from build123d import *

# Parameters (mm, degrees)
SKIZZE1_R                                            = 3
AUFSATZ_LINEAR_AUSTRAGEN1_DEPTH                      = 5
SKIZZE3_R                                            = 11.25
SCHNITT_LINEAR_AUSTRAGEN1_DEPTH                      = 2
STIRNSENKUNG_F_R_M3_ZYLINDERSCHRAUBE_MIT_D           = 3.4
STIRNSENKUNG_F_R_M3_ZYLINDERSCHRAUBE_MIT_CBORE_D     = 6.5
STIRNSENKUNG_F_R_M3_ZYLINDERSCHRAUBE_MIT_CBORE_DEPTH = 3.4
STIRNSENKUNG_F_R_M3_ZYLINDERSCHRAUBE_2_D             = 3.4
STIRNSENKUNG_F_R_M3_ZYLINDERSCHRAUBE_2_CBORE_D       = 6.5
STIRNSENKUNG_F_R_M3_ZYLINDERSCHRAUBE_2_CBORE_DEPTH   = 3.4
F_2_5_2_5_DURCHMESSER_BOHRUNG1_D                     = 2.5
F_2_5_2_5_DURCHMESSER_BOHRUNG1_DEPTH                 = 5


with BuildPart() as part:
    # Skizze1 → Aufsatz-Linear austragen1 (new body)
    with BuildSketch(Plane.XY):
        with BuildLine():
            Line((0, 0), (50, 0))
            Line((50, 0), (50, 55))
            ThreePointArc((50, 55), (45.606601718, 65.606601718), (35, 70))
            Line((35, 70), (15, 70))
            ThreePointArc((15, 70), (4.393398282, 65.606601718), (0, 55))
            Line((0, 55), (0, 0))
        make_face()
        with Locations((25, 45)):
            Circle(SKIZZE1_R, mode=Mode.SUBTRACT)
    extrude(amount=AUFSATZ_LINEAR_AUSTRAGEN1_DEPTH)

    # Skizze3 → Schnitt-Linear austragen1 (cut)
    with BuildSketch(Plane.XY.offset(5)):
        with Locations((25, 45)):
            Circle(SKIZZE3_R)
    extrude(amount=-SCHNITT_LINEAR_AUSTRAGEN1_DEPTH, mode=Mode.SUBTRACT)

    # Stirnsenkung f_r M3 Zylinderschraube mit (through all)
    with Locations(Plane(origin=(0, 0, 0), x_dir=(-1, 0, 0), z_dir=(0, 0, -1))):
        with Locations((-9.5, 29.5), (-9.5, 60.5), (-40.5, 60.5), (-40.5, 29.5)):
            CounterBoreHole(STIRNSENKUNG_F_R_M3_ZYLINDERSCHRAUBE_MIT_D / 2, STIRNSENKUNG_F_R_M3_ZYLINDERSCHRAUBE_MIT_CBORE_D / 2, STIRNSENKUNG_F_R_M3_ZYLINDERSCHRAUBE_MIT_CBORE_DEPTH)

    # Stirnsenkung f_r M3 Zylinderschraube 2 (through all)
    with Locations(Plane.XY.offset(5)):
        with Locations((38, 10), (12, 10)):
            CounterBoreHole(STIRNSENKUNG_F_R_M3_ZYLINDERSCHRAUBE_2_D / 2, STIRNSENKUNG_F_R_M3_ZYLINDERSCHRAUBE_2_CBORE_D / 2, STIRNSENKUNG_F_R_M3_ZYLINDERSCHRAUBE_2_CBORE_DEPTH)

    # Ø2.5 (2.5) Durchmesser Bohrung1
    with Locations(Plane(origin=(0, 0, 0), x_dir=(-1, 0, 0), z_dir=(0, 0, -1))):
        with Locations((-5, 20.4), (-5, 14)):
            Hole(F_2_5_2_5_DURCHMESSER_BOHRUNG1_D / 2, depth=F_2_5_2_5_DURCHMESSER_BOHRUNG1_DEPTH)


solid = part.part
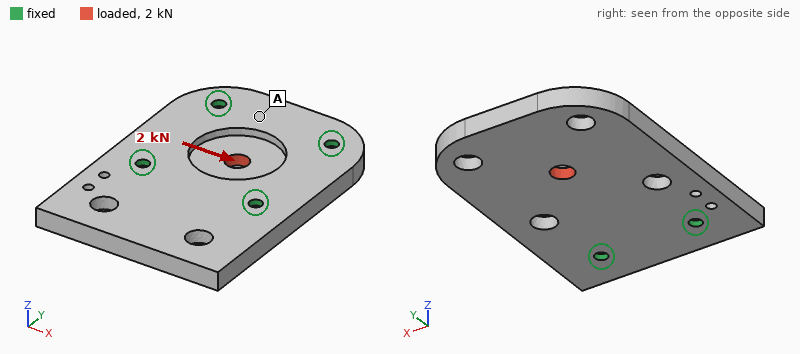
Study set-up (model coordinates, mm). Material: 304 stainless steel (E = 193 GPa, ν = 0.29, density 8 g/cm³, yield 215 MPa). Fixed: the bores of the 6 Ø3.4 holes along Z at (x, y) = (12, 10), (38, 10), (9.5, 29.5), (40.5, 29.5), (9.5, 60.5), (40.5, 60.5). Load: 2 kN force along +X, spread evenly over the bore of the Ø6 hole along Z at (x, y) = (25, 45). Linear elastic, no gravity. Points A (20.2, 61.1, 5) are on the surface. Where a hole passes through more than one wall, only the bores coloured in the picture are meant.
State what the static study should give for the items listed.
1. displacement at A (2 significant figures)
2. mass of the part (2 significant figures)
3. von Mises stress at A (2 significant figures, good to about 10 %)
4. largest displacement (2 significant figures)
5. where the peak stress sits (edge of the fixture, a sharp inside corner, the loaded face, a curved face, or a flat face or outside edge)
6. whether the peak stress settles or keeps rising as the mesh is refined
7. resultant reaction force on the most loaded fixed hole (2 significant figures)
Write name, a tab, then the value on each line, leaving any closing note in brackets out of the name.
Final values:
displacement at A	0.70 µm
mass of the part	120 g
von Mises stress at A	7.4 MPa
largest displacement	2.7 µm
where the peak stress sits	edge of the fixture
whether the peak stress settles or keeps rising as the mesh is refined	keeps rising
resultant reaction force on the most loaded fixed hole	510 N
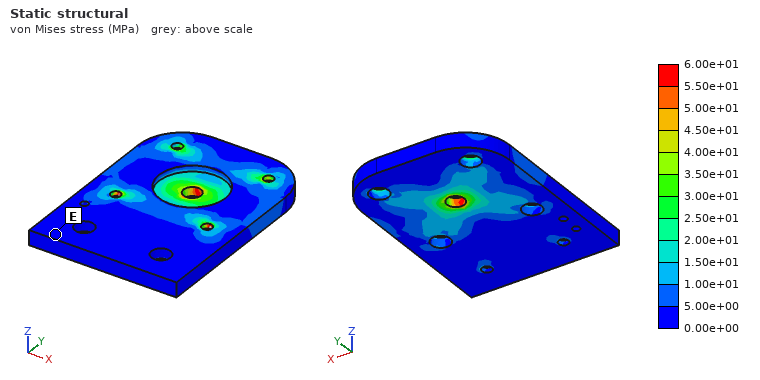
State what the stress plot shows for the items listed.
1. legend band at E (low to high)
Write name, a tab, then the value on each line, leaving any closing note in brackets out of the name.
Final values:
legend band at E	0.00e+00 to 5.00e+00 MPa
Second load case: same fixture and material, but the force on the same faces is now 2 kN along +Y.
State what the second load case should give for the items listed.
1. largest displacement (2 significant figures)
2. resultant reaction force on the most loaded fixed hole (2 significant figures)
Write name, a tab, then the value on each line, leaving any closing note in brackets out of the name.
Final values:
largest displacement	2.5 µm
resultant reaction force on the most loaded fixed hole	410 N
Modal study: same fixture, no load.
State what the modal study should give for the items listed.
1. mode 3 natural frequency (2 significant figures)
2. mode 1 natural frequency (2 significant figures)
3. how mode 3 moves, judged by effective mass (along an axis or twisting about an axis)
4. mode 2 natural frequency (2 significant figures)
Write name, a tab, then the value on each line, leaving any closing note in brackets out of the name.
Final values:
mode 3 natural frequency	15 kHz
mode 1 natural frequency	13 kHz
how mode 3 moves, judged by effective mass	twisting about Y
mode 2 natural frequency	14 kHz
